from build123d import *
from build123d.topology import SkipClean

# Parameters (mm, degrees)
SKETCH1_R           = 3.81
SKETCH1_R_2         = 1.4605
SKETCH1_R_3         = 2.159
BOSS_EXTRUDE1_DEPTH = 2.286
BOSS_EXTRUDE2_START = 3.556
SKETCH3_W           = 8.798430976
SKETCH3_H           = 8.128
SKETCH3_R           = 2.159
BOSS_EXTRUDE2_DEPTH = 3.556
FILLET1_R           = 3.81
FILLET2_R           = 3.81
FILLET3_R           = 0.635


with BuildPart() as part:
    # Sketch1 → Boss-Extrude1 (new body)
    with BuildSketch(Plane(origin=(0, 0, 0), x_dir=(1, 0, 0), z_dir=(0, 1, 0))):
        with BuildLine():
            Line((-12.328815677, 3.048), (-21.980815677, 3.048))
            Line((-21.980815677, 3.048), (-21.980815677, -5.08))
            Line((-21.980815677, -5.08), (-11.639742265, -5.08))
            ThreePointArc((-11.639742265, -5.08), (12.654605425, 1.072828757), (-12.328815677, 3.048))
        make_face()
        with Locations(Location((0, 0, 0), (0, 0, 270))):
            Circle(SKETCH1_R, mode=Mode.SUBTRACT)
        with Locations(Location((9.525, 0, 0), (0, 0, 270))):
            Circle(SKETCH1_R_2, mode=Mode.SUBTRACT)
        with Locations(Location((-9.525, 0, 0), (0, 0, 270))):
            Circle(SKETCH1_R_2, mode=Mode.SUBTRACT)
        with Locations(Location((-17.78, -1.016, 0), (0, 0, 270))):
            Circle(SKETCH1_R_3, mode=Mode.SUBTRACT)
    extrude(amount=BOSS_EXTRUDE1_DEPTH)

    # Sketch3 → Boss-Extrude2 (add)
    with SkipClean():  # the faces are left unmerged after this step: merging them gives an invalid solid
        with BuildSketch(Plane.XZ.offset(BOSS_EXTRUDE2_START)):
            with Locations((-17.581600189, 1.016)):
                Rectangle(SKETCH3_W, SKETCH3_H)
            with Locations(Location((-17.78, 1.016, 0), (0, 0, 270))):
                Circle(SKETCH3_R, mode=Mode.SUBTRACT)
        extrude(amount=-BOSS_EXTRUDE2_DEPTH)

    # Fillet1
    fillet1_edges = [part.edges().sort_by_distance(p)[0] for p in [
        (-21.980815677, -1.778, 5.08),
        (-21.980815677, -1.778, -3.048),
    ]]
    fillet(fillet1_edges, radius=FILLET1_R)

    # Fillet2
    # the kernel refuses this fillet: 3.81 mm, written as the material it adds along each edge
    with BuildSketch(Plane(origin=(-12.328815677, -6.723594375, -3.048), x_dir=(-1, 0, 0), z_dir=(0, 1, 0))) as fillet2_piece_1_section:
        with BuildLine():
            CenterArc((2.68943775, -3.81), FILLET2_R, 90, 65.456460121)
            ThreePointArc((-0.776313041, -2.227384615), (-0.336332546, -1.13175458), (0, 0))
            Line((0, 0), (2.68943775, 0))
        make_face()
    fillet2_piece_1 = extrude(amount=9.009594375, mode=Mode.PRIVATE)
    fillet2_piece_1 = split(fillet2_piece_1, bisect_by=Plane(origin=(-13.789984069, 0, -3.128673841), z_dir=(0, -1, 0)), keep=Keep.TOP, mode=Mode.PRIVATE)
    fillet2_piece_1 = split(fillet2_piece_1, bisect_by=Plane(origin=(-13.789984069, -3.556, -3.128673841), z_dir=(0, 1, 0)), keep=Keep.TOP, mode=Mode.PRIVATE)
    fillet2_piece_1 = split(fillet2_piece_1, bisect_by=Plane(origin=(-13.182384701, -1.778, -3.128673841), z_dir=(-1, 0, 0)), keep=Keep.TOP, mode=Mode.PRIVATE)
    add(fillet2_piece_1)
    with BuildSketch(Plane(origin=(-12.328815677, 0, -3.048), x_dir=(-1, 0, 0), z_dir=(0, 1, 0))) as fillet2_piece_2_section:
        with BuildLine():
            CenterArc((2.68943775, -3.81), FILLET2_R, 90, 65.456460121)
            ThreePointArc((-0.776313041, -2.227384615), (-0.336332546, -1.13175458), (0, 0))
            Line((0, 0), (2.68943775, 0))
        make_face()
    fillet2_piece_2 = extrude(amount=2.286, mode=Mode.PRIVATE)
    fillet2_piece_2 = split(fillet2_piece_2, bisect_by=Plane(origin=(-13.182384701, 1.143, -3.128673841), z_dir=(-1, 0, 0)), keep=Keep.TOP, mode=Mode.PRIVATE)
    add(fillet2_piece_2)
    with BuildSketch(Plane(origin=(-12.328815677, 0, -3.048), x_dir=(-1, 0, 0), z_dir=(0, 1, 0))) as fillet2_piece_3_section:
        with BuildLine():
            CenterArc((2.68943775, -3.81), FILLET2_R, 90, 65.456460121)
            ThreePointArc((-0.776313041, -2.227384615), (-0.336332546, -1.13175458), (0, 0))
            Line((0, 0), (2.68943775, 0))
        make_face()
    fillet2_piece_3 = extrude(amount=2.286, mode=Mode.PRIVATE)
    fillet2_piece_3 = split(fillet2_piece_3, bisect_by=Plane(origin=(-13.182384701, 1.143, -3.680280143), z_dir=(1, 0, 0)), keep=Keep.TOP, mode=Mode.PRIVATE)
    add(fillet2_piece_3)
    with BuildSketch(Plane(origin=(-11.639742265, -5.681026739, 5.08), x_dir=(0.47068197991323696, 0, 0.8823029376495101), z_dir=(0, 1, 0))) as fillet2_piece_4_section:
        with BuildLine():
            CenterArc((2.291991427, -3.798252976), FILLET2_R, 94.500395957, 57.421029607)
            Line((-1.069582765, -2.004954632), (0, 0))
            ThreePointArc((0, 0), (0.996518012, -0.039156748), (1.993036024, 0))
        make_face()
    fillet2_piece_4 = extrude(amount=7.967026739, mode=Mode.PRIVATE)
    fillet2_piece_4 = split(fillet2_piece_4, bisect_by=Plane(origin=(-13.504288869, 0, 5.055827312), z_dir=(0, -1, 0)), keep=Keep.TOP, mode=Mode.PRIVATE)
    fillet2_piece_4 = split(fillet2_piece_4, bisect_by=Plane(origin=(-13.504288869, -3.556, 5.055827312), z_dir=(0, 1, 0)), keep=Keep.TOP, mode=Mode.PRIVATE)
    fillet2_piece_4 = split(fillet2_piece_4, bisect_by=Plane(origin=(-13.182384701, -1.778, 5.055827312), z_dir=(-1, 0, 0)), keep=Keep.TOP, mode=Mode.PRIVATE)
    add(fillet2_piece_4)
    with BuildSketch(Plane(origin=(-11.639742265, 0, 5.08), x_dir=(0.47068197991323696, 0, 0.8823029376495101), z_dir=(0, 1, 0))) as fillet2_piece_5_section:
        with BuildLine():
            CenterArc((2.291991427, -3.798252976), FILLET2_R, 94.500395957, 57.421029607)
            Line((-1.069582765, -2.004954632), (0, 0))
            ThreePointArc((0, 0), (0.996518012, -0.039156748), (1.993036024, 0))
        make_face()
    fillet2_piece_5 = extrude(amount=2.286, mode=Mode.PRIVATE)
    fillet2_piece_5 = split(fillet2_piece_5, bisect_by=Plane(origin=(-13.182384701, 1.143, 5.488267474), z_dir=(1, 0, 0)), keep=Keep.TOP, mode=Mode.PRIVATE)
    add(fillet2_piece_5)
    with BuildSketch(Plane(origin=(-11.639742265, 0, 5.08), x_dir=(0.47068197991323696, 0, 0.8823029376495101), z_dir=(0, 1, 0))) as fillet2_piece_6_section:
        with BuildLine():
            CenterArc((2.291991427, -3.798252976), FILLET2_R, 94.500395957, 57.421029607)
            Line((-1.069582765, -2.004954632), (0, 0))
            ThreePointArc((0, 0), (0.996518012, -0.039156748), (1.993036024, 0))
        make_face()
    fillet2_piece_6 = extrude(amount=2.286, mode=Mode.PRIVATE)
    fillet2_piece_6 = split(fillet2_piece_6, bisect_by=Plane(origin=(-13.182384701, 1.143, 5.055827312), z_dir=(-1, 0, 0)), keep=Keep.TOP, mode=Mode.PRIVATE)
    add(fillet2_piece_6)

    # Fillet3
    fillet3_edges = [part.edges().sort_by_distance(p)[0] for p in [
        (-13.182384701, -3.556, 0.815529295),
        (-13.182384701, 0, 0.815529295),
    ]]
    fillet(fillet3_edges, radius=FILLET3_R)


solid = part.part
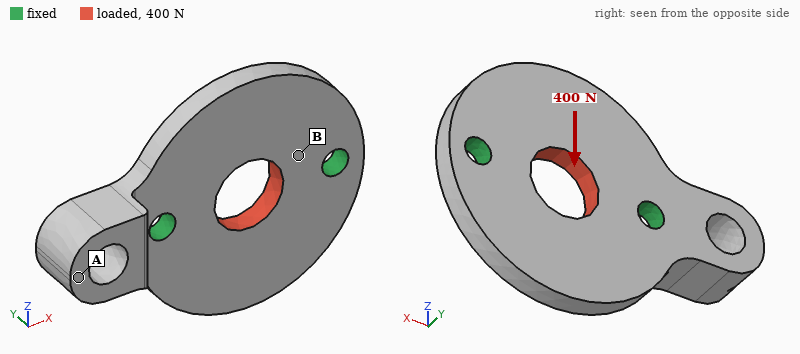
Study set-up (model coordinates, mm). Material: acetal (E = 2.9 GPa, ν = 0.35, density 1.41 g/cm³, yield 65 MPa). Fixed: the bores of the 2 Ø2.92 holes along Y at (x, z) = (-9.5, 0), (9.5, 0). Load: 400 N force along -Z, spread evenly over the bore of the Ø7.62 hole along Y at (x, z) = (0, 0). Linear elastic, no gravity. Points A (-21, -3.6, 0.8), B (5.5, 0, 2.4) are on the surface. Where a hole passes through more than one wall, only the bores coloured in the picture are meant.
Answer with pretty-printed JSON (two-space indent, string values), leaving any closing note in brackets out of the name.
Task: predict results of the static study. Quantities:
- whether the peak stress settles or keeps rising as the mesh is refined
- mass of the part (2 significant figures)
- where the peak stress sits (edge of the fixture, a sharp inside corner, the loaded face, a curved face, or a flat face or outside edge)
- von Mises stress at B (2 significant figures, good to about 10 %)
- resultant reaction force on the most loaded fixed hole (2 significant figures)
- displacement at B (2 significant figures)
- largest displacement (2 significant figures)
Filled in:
{
  "whether the peak stress settles or keeps rising as the mesh is refined": "keeps rising",
  "mass of the part": "1.9 g",
  "where the peak stress sits": "edge of the fixture",
  "von Mises stress at B": "9.1 MPa",
  "resultant reaction force on the most loaded fixed hole": "200 N",
  "displacement at B": "24 µm",
  "largest displacement": "43 µm"
}
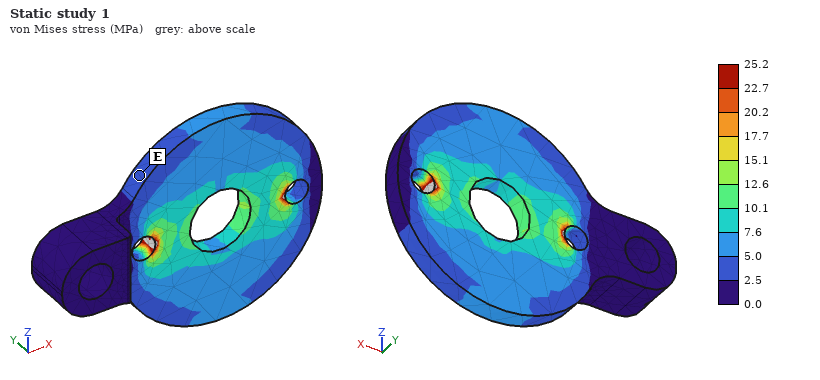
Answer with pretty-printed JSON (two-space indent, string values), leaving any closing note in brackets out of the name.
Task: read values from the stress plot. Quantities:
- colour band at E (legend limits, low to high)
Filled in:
{
  "colour band at E": "2.5 to 5.0 MPa"
}
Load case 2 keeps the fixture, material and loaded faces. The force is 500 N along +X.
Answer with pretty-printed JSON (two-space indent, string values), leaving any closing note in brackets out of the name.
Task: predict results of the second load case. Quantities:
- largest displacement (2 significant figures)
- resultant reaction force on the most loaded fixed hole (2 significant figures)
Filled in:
{
  "largest displacement": "39 µm",
  "resultant reaction force on the most loaded fixed hole": "260 N"
}
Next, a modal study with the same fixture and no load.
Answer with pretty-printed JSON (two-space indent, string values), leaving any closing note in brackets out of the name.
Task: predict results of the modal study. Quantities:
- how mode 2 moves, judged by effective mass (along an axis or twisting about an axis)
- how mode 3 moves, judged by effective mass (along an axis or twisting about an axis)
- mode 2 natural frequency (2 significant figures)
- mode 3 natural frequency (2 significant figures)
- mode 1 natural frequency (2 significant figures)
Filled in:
{
  "how mode 2 moves, judged by effective mass": "twisting about X",
  "how mode 3 moves, judged by effective mass": "along Y",
  "mode 2 natural frequency": "3400 Hz",
  "mode 3 natural frequency": "3900 Hz",
  "mode 1 natural frequency": "3200 Hz"
}
